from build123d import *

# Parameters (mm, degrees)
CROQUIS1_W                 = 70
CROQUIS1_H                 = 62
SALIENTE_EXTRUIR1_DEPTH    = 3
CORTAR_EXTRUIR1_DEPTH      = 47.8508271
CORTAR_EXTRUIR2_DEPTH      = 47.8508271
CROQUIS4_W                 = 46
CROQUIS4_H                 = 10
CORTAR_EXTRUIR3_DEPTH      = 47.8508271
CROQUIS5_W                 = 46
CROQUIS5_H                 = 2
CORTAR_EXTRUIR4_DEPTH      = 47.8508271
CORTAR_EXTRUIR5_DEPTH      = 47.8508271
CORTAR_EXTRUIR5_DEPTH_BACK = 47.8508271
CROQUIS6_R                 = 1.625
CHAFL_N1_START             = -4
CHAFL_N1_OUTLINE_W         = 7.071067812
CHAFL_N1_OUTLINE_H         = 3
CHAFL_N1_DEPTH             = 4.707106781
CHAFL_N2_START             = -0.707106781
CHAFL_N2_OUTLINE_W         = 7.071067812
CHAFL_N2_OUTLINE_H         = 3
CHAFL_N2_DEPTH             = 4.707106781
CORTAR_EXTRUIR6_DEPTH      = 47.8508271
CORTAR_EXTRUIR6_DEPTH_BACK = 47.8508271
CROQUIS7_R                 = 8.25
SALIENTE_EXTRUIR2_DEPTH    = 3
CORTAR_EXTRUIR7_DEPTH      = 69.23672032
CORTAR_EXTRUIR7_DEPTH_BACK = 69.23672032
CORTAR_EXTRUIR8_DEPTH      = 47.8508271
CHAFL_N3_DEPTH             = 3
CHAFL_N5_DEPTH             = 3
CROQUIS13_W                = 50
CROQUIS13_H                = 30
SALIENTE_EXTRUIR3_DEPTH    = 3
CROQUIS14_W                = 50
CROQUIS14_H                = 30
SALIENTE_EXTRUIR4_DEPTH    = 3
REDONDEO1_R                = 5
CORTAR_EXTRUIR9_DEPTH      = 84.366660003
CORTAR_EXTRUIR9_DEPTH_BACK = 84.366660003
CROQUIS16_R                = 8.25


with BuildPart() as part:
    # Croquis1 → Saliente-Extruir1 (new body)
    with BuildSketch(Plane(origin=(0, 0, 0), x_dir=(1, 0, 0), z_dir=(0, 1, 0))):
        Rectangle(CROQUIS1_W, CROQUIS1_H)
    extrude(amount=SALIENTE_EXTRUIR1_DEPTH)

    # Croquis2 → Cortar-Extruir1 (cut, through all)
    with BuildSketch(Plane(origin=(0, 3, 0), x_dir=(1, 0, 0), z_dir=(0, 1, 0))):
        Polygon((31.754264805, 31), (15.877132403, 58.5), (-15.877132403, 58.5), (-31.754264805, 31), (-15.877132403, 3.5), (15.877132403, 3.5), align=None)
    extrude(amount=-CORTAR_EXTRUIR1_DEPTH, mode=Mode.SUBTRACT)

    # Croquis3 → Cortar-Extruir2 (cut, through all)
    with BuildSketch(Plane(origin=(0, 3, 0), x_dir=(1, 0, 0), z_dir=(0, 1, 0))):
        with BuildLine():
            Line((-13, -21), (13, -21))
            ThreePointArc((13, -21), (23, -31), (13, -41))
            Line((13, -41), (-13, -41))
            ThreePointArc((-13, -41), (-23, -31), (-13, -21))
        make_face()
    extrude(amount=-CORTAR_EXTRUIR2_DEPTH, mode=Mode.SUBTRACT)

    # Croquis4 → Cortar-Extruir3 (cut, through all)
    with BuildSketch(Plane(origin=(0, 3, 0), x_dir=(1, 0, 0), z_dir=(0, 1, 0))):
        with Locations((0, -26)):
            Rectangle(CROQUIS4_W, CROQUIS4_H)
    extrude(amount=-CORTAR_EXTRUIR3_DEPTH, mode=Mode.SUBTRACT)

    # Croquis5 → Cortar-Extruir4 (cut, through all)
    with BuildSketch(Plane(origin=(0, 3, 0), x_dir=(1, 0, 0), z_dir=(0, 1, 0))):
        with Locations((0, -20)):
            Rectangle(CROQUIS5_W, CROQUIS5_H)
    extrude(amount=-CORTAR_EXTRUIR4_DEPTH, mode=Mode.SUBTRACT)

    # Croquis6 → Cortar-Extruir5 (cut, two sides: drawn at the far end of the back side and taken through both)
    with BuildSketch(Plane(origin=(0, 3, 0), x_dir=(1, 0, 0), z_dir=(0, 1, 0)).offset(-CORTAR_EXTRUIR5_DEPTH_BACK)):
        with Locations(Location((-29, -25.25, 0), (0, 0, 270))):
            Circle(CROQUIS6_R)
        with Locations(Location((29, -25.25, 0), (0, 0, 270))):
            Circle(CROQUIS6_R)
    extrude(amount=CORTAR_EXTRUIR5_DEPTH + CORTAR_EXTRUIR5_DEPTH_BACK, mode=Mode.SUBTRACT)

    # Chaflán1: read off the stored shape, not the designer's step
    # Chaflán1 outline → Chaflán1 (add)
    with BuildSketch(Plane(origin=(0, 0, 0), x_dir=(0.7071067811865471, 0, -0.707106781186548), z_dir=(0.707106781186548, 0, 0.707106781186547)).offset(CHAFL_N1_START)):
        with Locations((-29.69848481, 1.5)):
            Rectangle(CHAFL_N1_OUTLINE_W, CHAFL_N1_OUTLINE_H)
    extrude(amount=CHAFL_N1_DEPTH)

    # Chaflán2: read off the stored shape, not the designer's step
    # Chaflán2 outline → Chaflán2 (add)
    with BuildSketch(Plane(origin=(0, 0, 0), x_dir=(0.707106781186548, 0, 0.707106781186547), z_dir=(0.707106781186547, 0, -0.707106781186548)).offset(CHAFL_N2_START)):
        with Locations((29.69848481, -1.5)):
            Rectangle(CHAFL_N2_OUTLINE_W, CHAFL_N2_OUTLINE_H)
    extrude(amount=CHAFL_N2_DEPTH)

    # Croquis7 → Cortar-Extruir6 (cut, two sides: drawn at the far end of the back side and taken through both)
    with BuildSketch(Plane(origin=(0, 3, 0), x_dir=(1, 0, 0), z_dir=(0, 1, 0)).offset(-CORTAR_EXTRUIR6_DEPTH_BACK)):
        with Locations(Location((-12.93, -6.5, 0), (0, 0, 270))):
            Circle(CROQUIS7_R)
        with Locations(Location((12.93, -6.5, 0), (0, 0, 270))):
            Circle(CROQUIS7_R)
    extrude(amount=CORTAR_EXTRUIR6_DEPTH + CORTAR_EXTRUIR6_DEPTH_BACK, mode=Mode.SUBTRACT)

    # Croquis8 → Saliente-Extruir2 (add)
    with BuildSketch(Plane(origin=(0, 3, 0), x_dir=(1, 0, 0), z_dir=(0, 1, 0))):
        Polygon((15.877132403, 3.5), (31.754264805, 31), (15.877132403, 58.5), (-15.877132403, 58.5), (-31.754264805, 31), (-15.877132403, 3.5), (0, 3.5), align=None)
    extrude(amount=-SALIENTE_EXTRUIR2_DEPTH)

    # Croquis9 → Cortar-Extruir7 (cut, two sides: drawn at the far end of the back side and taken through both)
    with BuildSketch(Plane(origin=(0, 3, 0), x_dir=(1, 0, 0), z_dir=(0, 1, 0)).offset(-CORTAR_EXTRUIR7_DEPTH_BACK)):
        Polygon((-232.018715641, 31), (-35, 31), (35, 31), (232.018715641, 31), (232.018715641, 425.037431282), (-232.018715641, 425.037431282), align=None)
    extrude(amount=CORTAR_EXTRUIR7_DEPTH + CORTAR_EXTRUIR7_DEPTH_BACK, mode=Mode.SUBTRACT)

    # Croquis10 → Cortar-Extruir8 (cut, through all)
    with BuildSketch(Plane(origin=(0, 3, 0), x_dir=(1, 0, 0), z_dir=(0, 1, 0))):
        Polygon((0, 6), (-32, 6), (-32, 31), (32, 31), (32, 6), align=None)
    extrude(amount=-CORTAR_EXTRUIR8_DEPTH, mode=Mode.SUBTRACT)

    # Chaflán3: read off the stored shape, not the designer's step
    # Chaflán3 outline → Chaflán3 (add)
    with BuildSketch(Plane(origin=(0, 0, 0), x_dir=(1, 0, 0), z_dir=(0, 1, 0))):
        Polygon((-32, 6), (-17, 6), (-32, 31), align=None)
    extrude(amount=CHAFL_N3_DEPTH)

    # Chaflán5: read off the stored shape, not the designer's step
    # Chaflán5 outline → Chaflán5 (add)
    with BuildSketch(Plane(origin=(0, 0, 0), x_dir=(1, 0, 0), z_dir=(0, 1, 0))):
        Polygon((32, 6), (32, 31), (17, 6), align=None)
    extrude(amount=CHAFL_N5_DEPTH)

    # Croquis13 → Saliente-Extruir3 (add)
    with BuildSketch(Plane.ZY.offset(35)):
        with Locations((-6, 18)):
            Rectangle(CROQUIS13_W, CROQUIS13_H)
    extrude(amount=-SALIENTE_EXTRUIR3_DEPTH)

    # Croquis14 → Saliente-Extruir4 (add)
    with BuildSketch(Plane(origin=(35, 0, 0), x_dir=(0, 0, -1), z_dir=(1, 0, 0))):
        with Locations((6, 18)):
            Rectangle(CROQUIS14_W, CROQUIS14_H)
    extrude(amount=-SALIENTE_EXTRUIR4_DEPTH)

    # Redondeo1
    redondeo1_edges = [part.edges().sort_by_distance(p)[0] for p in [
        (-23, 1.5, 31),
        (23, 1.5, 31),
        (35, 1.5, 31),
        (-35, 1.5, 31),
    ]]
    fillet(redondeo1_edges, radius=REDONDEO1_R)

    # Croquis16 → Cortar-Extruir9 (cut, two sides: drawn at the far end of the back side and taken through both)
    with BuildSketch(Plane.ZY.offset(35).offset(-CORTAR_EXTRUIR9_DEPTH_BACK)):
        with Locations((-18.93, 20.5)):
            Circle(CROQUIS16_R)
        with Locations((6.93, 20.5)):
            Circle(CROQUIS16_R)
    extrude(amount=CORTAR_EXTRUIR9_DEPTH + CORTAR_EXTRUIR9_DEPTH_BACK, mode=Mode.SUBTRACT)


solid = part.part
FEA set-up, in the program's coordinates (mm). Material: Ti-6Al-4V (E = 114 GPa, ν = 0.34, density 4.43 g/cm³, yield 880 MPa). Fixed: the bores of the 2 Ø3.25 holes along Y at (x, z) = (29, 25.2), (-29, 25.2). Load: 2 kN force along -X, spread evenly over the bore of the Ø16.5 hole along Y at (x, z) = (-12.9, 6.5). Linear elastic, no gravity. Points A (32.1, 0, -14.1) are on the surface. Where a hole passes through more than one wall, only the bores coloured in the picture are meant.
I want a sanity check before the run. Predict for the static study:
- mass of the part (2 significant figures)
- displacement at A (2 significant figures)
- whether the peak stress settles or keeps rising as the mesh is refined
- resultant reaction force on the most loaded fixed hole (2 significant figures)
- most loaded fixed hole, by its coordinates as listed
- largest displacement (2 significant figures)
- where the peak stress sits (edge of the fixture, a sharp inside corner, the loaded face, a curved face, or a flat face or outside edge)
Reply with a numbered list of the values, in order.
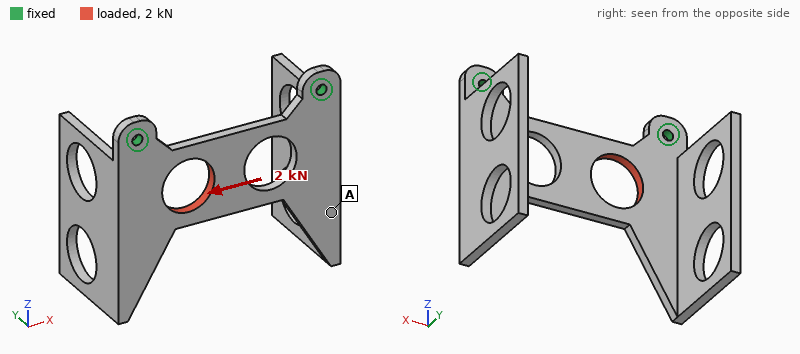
1. 57 g
2. 36 µm
3. keeps rising
4. 1.2 kN
5. (-29, 25.2)
6. 60 µm
7. edge of the fixture
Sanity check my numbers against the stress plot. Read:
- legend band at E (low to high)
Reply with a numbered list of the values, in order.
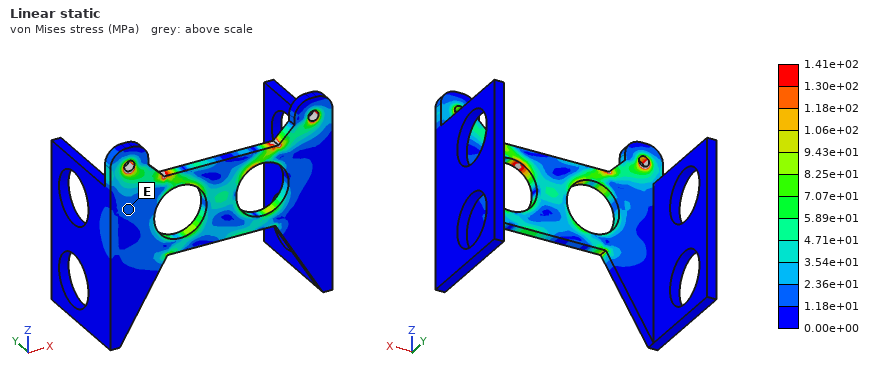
1. 1.18e+01 to 2.36e+01 MPa
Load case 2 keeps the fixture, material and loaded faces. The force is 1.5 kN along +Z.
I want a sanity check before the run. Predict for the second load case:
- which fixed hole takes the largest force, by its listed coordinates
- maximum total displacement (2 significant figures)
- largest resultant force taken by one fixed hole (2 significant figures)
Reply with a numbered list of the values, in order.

1. (-29, 25.2)
2. 25 µm
3. 1.2 kN
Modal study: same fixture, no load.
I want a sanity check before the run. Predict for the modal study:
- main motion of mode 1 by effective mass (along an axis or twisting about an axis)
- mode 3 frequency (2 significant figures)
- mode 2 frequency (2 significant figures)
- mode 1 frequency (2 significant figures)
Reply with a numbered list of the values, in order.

1. along Y
2. 1200 Hz
3. 720 Hz
4. 610 Hz
